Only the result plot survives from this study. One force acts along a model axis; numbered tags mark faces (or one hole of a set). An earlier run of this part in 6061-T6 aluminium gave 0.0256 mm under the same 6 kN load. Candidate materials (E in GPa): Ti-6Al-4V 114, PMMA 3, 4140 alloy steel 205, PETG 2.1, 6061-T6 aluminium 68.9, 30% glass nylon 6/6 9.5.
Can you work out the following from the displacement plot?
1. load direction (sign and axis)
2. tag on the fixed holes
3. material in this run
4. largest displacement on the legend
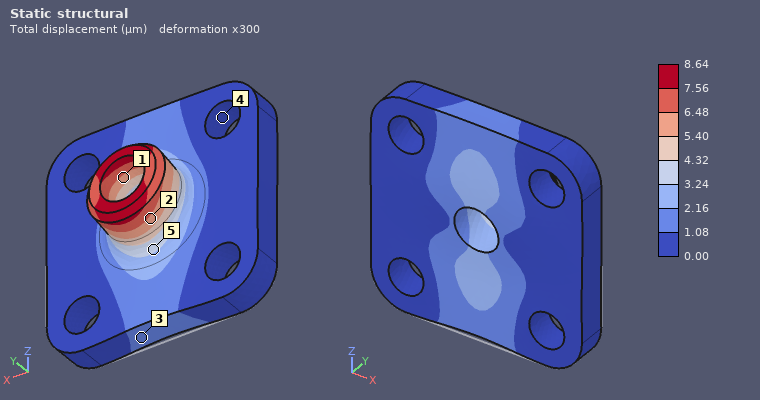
+Z
4
4140 alloy steel
8.64 µm
